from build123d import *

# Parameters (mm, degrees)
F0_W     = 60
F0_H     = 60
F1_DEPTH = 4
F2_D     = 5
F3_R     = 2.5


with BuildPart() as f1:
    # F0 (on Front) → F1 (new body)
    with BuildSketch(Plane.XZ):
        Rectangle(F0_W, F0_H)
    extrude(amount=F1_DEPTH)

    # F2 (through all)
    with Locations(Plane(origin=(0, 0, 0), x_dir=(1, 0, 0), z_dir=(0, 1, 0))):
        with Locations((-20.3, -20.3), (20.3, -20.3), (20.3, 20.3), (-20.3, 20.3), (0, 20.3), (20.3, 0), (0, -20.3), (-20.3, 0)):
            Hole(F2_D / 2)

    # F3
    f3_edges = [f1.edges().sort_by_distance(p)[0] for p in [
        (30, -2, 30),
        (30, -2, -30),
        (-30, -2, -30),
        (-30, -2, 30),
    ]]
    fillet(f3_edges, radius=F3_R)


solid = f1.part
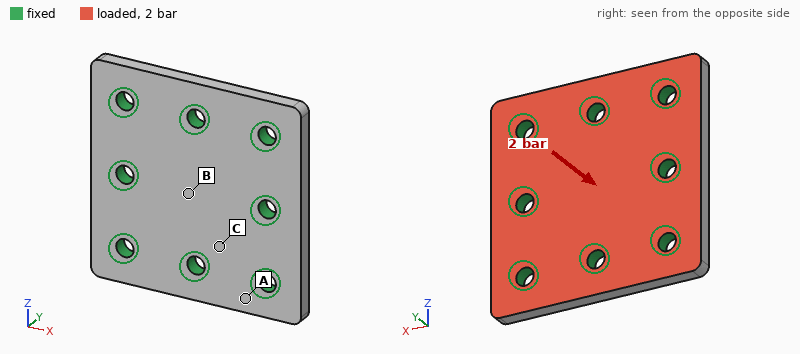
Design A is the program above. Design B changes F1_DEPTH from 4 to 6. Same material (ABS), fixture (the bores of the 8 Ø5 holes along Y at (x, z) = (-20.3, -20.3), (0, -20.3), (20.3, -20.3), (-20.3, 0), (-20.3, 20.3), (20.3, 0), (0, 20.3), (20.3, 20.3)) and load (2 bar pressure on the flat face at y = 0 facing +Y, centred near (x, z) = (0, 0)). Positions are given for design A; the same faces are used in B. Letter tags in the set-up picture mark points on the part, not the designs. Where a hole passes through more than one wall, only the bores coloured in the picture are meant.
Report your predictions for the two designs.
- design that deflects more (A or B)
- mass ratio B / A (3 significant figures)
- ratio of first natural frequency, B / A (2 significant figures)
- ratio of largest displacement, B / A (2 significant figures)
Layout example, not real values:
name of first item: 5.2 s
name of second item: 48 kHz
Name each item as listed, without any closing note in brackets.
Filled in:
design that deflects more: A
mass ratio B / A: 1.50
ratio of first natural frequency, B / A: 1.3
ratio of largest displacement, B / A: 0.37
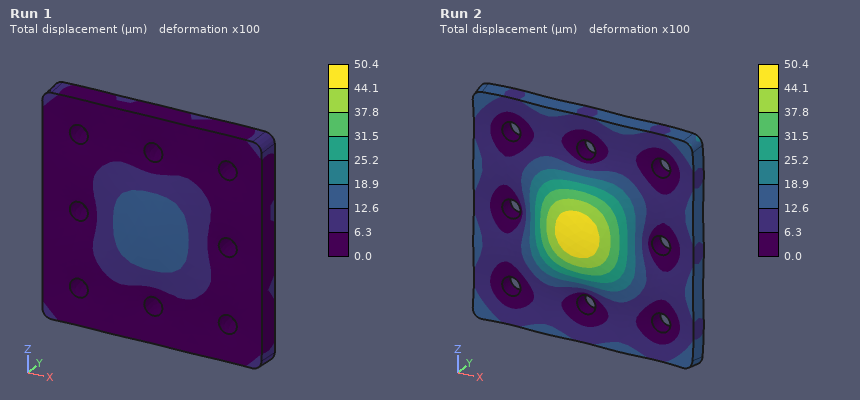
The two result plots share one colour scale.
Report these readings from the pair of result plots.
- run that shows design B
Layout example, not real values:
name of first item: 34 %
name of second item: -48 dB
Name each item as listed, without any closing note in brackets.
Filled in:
run that shows design B: Run 1
